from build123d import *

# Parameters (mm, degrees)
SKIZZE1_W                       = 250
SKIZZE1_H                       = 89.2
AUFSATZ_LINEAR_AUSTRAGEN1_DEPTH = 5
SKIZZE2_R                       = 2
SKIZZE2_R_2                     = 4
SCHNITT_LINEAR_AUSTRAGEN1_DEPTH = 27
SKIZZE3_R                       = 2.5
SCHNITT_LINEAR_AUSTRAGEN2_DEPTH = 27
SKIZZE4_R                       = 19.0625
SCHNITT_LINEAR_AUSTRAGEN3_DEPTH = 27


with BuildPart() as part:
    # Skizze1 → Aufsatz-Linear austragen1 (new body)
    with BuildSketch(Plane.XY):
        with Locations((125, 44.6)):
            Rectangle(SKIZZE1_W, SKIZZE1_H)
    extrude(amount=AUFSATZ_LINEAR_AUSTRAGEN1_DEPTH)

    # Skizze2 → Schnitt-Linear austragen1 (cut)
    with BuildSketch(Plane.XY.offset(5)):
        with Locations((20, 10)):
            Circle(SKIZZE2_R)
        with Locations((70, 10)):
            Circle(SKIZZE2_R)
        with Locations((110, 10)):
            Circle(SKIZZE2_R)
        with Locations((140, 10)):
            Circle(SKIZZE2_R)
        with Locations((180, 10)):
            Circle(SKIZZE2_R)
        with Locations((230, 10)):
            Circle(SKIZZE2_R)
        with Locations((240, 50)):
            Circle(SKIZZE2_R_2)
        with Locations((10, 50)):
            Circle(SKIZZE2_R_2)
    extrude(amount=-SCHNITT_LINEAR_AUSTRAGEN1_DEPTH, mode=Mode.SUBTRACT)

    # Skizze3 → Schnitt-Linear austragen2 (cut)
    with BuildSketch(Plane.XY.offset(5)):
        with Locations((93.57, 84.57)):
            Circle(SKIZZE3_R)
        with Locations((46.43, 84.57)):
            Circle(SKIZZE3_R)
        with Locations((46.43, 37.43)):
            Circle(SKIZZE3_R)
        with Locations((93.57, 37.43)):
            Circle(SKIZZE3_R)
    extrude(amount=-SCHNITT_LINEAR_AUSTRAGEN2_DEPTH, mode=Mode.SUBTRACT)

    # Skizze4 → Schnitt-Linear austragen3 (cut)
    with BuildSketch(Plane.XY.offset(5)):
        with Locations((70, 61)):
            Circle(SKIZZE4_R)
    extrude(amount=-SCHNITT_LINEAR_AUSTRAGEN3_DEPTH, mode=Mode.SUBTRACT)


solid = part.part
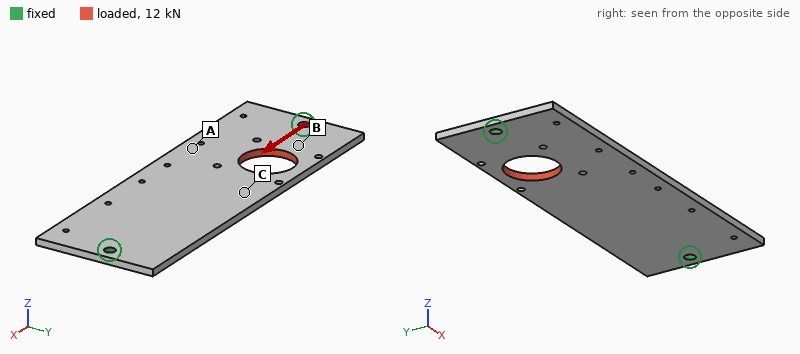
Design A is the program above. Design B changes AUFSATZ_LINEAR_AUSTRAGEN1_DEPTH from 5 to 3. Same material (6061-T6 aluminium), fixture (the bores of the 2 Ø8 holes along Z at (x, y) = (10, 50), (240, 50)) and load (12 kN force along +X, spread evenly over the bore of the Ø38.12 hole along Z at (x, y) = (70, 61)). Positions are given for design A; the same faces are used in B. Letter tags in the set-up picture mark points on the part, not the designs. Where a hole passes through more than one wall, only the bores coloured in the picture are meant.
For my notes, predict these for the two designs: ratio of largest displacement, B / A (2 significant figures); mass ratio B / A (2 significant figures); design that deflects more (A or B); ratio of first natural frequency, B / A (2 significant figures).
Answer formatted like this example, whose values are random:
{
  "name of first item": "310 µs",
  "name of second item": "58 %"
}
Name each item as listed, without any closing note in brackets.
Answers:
{
  "ratio of largest displacement, B / A": "1.7",
  "mass ratio B / A": "0.60",
  "design that deflects more": "B",
  "ratio of first natural frequency, B / A": "0.61"
}
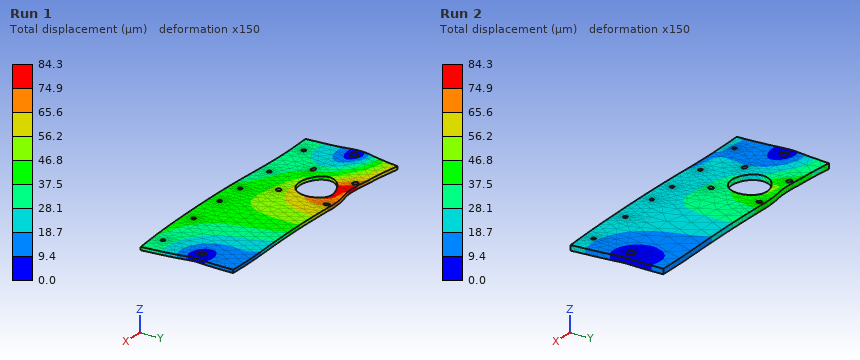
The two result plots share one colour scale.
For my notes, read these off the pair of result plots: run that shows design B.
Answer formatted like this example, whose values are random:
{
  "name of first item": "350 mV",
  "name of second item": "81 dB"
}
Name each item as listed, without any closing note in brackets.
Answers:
{
  "run that shows design B": "Run 1"
}
